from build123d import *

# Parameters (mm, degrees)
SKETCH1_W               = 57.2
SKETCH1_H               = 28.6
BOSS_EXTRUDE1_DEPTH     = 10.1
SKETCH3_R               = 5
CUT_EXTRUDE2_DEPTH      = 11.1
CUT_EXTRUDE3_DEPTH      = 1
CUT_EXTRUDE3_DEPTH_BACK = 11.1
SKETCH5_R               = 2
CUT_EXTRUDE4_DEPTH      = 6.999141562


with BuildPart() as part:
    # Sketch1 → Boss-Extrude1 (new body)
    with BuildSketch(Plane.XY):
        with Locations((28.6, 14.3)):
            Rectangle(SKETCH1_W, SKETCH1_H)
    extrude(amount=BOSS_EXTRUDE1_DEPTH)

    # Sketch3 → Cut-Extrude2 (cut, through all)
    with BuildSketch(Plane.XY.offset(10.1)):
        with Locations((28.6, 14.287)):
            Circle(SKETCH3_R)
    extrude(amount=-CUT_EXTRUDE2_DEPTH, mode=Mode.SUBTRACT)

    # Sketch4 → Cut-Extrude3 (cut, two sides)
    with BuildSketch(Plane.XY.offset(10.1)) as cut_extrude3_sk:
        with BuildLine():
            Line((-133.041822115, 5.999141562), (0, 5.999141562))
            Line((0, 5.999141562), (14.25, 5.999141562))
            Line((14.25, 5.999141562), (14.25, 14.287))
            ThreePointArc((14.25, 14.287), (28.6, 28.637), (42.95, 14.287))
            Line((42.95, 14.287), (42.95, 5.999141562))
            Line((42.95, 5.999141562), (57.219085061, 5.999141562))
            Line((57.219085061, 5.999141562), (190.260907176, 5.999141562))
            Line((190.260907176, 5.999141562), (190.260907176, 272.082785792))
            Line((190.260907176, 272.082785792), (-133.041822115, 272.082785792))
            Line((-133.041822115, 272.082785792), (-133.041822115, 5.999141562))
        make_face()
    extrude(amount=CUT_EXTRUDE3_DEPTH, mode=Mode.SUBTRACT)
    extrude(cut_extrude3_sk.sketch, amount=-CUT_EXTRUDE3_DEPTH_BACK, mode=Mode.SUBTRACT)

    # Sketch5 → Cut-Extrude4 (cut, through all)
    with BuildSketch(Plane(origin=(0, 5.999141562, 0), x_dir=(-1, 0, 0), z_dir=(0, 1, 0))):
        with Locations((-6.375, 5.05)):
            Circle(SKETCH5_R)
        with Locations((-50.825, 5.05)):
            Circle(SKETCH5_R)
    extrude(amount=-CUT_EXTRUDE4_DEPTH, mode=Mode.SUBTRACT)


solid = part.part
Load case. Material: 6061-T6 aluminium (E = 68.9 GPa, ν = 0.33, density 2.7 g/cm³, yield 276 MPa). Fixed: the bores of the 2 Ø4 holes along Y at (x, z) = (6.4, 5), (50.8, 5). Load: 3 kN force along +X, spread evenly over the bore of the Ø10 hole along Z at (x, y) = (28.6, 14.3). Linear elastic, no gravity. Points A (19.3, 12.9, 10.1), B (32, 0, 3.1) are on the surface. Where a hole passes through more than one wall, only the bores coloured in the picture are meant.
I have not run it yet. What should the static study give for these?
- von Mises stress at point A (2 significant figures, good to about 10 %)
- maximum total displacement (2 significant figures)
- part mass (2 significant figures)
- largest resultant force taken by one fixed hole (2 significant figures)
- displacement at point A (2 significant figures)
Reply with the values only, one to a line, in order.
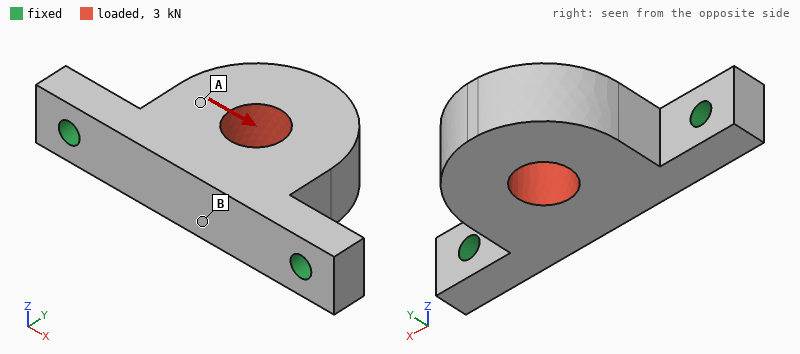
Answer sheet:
25 MPa
27 µm
22 g
1.8 kN
14 µm
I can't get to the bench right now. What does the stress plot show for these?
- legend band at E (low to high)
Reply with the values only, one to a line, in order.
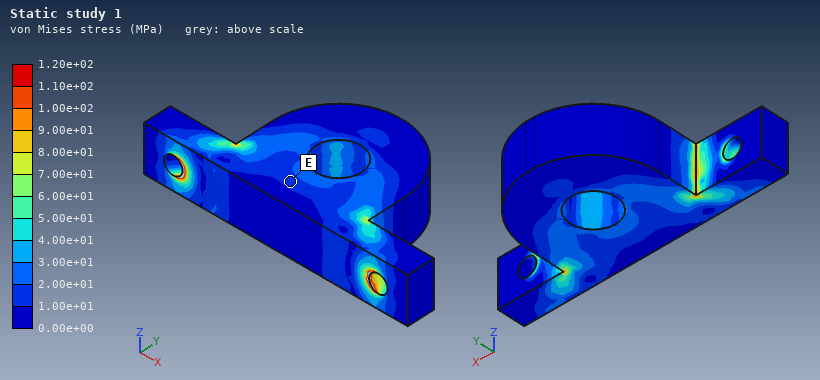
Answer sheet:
1.00e+01 to 2.00e+01 MPa
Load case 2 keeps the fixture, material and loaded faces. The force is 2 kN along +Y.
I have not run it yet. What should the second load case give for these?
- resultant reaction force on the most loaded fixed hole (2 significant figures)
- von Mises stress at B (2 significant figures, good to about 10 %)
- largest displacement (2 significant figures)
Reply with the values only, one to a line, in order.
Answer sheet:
1.1 kN
17 MPa
18 µm
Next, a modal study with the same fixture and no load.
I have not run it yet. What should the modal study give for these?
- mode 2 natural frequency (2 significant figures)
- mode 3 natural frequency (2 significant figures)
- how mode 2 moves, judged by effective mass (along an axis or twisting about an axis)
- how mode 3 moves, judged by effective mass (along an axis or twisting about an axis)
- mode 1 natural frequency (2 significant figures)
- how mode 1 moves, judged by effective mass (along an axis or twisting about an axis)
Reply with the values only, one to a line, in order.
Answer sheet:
14 kHz
15 kHz
along Y
along X
4500 Hz
along Z
